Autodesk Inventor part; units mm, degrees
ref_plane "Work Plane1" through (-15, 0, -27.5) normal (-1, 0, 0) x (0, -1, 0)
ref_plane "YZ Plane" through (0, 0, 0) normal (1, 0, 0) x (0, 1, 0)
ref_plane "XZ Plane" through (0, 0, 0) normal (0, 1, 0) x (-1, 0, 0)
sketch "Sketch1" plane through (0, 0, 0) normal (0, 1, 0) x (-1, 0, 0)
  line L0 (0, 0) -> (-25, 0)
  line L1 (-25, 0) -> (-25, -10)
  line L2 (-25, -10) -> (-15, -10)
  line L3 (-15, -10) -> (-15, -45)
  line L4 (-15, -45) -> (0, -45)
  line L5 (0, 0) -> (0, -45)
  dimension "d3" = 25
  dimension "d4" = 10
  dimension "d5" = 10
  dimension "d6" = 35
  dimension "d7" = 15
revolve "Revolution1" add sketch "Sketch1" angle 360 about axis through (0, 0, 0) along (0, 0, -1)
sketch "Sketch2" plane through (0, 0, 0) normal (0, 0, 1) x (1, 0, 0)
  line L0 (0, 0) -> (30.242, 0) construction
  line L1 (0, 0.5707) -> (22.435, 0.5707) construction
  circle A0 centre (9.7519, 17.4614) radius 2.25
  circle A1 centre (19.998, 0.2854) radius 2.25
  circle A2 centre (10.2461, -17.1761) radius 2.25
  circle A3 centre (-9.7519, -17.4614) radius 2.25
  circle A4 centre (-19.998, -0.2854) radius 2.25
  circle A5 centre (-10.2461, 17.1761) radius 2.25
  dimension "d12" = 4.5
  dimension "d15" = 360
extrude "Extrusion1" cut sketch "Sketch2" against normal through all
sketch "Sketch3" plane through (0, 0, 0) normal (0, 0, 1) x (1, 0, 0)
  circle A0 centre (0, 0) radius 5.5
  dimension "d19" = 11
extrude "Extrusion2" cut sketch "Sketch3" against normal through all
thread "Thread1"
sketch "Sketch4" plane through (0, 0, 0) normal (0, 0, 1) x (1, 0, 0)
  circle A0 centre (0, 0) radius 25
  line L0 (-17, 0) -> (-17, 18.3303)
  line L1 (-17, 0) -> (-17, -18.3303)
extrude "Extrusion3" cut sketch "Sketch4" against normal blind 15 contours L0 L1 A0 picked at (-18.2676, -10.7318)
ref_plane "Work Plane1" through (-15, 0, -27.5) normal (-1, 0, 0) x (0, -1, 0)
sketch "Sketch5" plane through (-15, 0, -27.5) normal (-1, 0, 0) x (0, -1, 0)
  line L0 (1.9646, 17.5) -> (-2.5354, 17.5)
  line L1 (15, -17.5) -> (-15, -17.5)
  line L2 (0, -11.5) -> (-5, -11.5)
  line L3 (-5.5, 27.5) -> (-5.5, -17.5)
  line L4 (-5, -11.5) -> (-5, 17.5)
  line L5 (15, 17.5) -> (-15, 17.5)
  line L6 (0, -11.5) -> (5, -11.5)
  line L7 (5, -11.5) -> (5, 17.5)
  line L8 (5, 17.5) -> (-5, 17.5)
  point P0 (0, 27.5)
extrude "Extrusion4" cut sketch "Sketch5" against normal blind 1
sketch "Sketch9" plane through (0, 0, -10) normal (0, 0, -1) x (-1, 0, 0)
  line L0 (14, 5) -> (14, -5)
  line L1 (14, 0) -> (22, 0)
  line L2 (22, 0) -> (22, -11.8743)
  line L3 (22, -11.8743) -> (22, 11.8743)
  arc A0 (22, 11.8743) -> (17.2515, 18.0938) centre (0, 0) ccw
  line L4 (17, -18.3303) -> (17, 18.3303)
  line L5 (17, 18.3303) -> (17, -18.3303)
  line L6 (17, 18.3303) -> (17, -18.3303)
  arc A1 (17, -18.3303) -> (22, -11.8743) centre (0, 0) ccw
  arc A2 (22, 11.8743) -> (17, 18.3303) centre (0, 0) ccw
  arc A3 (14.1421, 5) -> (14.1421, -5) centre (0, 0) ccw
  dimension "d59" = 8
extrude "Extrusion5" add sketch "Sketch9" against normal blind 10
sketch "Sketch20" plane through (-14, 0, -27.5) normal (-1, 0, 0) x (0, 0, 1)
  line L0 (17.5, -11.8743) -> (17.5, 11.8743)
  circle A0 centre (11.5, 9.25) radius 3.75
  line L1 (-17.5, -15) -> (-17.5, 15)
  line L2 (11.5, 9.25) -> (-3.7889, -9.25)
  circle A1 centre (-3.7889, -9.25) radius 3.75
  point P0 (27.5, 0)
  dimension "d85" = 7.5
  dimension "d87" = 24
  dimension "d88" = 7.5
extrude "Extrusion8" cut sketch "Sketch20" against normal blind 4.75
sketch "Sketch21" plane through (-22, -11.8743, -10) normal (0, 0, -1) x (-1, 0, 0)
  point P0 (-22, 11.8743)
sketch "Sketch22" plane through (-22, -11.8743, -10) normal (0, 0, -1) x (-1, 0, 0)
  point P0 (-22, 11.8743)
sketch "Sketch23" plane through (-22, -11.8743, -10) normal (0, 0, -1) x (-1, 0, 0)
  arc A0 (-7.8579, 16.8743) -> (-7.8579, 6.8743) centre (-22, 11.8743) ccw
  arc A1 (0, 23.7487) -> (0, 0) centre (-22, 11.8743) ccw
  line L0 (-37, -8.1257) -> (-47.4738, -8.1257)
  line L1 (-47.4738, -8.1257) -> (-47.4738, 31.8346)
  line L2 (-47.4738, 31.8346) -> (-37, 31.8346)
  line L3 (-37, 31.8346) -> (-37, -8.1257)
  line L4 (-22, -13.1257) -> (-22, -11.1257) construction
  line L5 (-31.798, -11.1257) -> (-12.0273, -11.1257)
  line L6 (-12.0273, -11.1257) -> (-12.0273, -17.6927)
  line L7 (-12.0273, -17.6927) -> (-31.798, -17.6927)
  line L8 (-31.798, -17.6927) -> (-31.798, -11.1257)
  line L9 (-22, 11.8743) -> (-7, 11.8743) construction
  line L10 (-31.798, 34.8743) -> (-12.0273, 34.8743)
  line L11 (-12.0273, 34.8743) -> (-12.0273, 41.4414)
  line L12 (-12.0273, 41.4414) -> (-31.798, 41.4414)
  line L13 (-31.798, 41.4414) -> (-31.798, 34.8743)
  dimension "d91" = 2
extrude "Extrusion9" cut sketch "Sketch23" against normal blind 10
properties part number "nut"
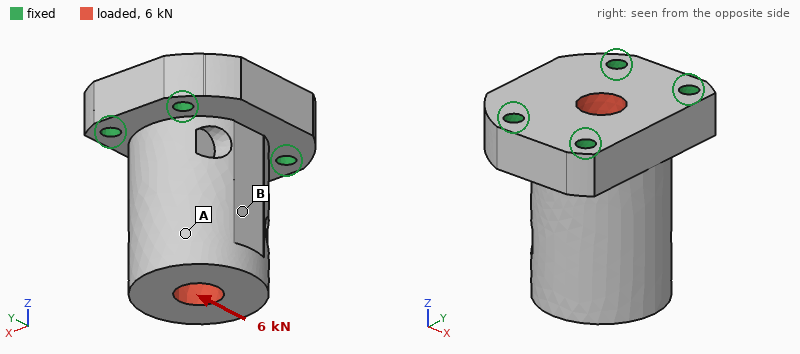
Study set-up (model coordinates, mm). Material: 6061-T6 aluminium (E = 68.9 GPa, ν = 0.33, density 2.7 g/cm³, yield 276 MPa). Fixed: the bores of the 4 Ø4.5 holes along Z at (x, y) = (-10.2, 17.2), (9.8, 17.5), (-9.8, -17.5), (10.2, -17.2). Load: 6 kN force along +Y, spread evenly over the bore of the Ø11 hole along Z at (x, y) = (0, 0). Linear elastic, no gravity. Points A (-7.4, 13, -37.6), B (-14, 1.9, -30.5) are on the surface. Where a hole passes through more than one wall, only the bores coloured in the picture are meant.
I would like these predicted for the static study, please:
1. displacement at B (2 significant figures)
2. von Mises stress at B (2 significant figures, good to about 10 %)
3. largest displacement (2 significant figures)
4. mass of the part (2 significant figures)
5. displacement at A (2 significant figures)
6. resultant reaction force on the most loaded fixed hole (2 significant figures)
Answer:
18 µm
9.7 MPa
31 µm
95 g
25 µm
2.3 kN
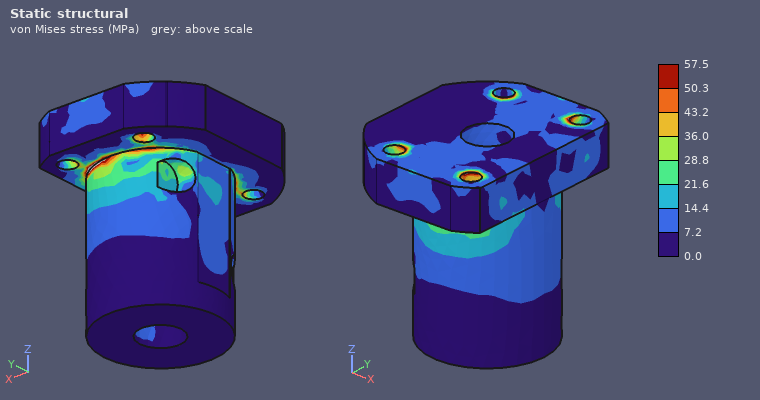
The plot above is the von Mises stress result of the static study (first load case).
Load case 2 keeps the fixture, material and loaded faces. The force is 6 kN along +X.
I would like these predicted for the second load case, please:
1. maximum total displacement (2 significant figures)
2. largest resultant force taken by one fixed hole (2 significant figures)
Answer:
53 µm
2.9 kN
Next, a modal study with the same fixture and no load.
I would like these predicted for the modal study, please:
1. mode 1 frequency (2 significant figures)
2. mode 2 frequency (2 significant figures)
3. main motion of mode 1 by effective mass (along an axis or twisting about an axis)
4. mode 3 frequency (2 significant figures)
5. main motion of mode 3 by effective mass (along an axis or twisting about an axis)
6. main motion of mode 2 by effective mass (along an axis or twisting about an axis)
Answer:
7400 Hz
9800 Hz
along X
19 kHz
along Z
along Y
